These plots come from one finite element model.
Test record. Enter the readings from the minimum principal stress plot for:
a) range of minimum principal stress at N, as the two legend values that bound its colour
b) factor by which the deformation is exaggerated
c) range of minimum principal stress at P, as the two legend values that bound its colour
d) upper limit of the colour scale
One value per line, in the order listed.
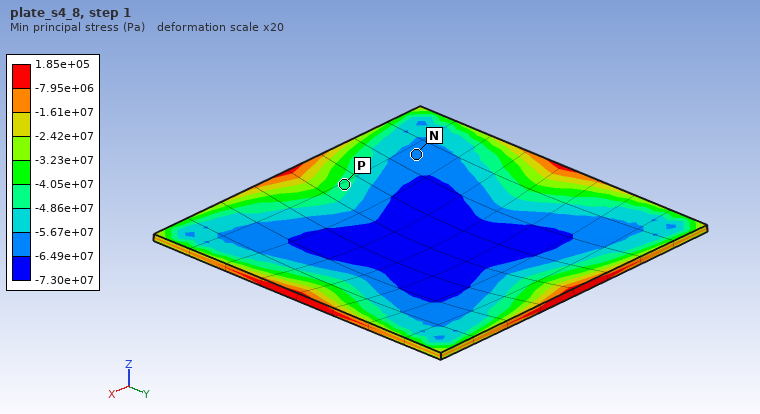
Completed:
-6.49e+07 to -5.67e+07 Pa
20
-4.86e+07 to -4.05e+07 Pa
1.85e+05 Pa
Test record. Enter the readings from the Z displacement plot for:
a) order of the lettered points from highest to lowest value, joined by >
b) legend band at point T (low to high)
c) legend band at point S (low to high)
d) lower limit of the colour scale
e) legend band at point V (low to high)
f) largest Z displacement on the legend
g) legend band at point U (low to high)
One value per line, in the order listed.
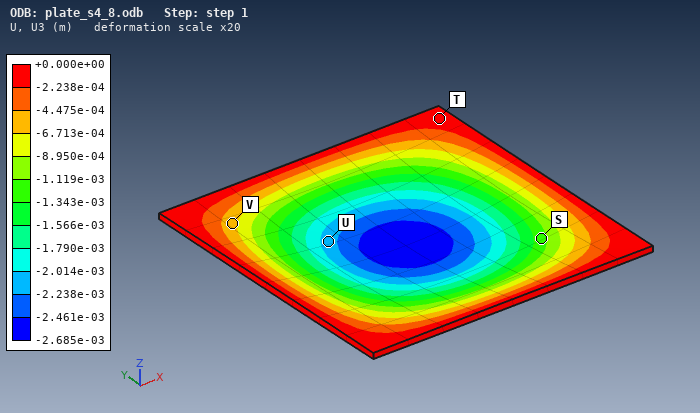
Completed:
T > V > S > U
-2.238e-04 to +0.000e+00 m
-1.343e-03 to -1.119e-03 m
-2.685e-03 m
-6.713e-04 to -4.475e-04 m
+0.000e+00 m
-2.238e-03 to -2.014e-03 m
